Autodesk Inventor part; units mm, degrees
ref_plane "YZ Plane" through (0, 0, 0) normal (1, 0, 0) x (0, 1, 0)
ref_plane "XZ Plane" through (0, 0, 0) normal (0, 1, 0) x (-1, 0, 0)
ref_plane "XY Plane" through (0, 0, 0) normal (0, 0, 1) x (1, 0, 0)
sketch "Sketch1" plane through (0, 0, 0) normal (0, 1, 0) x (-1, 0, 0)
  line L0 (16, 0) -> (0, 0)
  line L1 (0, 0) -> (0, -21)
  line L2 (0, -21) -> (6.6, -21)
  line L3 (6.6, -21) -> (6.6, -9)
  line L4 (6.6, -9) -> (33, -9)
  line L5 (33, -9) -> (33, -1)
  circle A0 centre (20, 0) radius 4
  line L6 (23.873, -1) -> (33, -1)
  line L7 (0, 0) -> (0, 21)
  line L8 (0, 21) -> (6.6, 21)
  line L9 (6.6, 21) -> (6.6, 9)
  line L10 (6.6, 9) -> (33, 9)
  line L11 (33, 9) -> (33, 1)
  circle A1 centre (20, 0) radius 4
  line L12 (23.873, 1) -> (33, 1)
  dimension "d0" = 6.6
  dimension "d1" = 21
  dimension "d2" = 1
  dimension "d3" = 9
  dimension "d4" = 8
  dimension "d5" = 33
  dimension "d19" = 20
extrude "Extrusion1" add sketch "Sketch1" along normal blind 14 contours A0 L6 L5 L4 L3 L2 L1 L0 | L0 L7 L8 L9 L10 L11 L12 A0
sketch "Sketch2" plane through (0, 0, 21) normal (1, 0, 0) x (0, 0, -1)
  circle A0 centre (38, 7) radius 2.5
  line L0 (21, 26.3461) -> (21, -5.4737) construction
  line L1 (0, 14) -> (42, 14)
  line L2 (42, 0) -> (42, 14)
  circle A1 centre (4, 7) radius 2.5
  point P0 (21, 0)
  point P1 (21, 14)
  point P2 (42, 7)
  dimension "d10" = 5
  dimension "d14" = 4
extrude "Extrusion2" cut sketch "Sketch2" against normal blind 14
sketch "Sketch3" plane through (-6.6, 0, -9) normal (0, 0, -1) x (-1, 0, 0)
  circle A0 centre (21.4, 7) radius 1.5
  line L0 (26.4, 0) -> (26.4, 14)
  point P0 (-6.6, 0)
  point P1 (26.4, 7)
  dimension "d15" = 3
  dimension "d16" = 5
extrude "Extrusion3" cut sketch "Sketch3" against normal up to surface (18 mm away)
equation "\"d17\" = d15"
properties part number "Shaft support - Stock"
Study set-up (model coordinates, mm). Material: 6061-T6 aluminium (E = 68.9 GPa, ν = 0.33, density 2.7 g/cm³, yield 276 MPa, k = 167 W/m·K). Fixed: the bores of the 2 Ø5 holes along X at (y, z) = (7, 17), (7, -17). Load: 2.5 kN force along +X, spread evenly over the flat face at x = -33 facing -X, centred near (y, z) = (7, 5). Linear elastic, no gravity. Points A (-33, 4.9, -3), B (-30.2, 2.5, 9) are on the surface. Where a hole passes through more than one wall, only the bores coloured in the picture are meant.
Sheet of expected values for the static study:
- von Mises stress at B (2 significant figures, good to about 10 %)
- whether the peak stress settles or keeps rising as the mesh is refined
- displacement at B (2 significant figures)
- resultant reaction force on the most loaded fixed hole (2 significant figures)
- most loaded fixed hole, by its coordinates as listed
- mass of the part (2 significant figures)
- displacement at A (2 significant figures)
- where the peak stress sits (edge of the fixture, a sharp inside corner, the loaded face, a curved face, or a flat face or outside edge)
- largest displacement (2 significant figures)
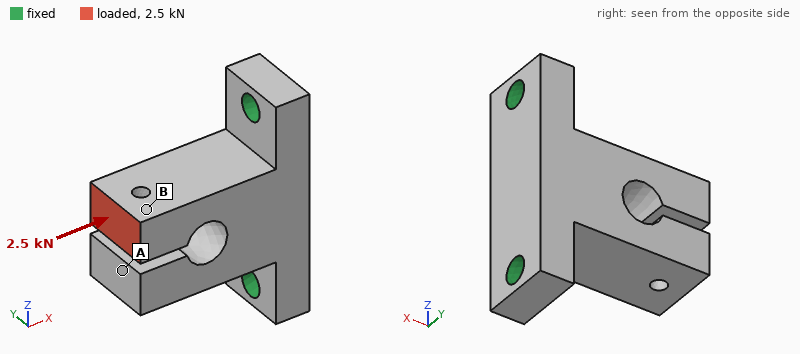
24 MPa
keeps rising
20 µm
1.8 kN
(7, 17)
25 g
16 µm
edge of the fixture
37 µm
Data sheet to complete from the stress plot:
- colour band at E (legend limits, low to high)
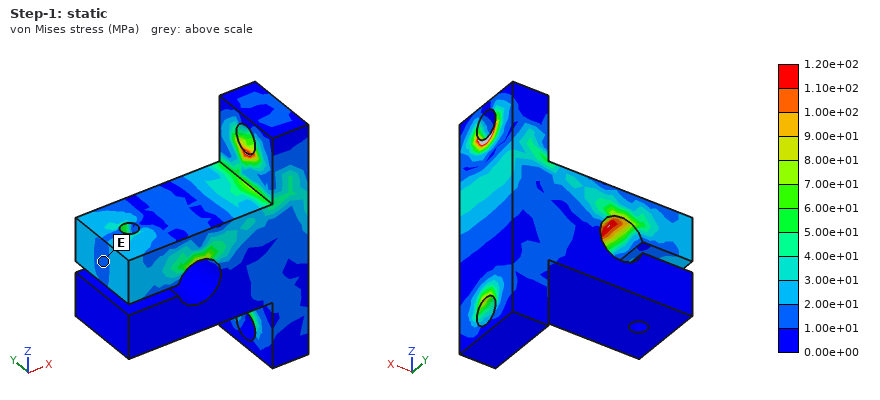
1.00e+01 to 2.00e+01 MPa
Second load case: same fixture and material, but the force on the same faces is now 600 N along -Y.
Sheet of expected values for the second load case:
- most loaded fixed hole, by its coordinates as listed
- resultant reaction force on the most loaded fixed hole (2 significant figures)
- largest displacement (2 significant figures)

(7, 17)
390 N
0.13 mm
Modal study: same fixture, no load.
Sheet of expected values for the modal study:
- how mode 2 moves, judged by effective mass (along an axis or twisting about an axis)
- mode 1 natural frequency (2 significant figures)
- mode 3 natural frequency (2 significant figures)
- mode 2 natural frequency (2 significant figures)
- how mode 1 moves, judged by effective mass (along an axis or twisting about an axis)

along Z
5100 Hz
9900 Hz
8200 Hz
along Y
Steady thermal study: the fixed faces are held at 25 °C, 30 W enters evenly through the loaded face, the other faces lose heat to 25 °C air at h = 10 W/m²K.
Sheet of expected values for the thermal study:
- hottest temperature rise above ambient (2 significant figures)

58 K
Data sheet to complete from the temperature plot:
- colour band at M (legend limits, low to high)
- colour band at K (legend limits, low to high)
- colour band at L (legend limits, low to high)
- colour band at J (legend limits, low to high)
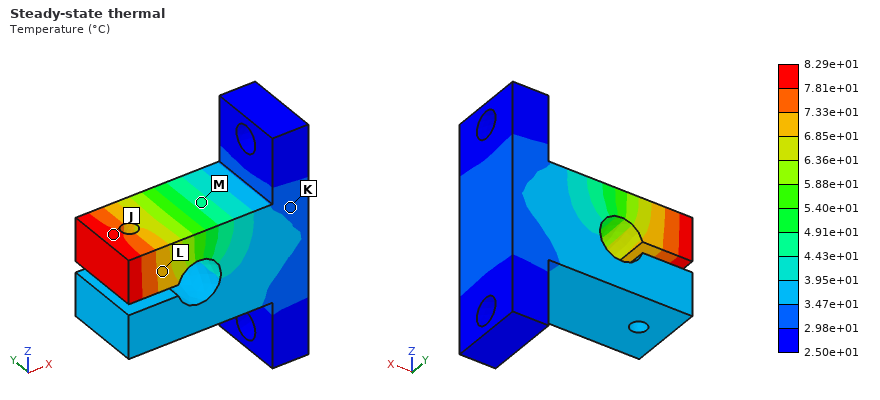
4.43e+01 to 4.91e+01 °C
2.98e+01 to 3.47e+01 °C
6.85e+01 to 7.33e+01 °C
7.81e+01 to 8.29e+01 °C
